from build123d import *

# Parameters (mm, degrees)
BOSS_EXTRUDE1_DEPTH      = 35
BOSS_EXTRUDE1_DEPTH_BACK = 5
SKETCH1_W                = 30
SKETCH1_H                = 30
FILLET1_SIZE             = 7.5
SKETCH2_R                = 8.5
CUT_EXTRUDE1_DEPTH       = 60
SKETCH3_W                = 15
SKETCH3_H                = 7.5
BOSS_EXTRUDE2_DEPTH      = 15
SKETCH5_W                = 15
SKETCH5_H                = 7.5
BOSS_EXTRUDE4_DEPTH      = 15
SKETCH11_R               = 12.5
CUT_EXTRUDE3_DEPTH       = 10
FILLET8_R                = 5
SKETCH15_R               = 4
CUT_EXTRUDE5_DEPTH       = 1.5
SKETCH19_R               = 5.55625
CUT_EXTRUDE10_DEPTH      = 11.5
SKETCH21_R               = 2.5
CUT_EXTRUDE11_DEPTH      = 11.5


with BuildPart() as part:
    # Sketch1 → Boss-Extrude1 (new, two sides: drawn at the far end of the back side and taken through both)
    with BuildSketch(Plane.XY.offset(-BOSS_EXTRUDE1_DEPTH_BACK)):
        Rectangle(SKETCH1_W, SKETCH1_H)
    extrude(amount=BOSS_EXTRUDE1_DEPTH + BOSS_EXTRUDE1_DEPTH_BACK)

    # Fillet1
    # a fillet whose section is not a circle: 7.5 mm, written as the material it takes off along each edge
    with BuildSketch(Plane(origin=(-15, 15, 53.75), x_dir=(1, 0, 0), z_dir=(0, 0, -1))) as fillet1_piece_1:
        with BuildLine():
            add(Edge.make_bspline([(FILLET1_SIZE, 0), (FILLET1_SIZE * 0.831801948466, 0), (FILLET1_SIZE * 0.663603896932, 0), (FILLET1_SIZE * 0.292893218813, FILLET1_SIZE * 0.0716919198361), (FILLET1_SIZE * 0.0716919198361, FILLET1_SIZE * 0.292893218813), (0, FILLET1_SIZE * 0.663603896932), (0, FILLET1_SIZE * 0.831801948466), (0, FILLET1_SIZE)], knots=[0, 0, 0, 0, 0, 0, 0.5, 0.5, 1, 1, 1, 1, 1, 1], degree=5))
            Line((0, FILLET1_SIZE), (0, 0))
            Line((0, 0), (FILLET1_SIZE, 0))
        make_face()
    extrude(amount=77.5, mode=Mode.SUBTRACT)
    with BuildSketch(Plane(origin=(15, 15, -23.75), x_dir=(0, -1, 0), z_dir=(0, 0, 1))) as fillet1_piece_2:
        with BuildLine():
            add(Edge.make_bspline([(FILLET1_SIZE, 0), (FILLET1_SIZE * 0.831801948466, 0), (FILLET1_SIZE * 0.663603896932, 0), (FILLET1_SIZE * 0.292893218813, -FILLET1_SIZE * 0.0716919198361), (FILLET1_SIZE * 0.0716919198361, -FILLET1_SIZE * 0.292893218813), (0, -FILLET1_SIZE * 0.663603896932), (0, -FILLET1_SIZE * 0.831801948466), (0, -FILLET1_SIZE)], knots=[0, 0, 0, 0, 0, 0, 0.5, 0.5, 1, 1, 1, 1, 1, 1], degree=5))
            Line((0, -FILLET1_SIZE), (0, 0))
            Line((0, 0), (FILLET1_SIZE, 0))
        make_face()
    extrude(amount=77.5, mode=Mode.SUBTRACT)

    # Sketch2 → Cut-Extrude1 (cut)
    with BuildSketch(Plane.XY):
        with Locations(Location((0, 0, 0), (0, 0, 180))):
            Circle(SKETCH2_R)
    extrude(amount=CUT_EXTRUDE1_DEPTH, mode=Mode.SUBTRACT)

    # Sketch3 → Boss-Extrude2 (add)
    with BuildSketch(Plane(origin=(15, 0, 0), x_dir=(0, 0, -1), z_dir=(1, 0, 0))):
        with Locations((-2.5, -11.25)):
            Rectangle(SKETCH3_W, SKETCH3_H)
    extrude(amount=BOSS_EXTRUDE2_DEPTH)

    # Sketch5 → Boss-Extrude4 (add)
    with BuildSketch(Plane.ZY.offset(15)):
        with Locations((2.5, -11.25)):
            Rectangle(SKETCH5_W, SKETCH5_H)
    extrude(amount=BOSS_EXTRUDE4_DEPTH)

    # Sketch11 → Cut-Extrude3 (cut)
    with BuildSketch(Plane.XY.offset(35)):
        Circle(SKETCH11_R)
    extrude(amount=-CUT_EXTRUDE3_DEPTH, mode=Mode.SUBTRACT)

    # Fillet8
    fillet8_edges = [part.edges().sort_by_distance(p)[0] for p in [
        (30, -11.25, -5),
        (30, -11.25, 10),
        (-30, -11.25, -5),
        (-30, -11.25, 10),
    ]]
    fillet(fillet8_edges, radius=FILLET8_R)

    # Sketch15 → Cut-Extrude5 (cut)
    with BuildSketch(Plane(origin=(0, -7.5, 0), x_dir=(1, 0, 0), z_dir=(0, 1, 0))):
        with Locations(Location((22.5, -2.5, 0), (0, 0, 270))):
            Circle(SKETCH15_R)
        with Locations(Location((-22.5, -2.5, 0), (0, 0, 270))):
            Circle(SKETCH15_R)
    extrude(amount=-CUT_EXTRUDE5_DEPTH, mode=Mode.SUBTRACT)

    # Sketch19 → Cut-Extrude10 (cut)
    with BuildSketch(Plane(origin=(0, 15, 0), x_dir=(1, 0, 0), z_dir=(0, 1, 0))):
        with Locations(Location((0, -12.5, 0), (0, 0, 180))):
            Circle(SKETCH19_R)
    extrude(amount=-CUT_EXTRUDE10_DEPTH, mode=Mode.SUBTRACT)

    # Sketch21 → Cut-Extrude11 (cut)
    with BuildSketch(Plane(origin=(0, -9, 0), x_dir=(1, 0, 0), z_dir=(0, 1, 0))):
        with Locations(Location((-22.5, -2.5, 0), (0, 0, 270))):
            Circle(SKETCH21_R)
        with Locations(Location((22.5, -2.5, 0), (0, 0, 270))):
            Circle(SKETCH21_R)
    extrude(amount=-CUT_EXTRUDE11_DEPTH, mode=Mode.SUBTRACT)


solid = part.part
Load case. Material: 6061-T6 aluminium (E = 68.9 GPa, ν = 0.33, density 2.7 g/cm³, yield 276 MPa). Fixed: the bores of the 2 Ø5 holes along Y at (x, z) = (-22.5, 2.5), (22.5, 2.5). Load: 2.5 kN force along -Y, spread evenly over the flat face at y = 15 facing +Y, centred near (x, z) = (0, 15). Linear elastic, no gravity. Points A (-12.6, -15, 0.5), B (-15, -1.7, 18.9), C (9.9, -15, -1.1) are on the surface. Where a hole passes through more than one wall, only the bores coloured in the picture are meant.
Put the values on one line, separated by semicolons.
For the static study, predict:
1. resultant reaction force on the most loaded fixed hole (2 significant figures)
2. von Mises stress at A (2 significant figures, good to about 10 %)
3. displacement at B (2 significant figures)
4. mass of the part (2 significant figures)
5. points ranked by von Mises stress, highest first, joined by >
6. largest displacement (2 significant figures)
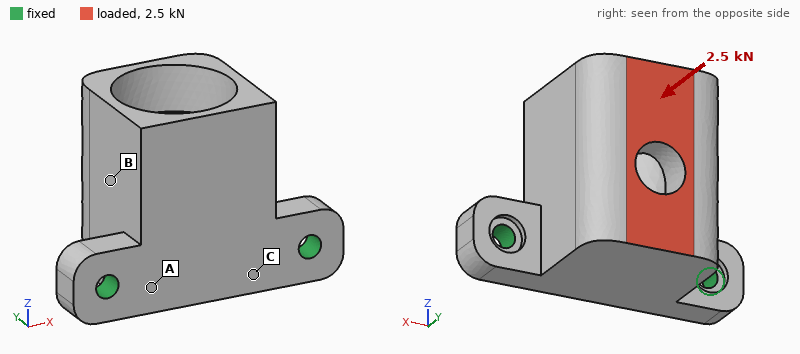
1.4 kN; 50 MPa; 0.090 mm; 73 g; A > C > B; 0.21 mm
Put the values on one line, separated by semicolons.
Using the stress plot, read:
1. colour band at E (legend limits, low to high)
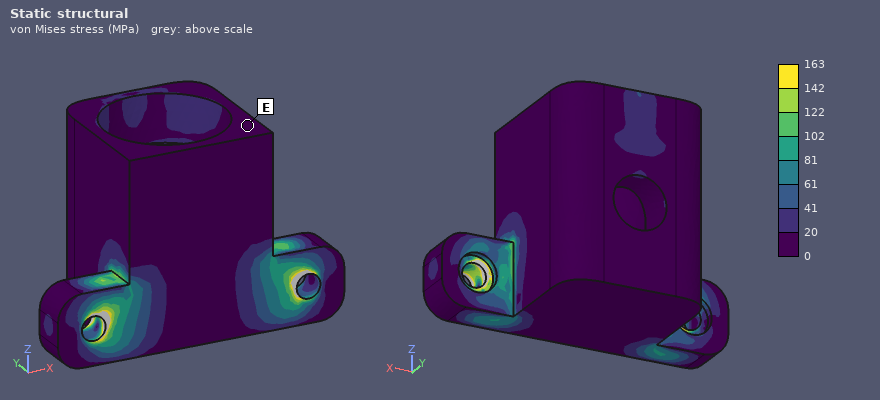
0 to 20 MPa
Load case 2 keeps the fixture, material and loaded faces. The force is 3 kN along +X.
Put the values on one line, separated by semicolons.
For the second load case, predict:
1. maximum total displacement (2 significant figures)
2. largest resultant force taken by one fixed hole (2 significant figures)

56 µm; 2.8 kN
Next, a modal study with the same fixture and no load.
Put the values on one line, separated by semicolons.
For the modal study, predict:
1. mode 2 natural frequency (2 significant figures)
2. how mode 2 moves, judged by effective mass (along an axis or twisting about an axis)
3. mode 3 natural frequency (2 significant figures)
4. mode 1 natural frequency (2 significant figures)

8500 Hz; along X; 10 kHz; 2500 Hz
